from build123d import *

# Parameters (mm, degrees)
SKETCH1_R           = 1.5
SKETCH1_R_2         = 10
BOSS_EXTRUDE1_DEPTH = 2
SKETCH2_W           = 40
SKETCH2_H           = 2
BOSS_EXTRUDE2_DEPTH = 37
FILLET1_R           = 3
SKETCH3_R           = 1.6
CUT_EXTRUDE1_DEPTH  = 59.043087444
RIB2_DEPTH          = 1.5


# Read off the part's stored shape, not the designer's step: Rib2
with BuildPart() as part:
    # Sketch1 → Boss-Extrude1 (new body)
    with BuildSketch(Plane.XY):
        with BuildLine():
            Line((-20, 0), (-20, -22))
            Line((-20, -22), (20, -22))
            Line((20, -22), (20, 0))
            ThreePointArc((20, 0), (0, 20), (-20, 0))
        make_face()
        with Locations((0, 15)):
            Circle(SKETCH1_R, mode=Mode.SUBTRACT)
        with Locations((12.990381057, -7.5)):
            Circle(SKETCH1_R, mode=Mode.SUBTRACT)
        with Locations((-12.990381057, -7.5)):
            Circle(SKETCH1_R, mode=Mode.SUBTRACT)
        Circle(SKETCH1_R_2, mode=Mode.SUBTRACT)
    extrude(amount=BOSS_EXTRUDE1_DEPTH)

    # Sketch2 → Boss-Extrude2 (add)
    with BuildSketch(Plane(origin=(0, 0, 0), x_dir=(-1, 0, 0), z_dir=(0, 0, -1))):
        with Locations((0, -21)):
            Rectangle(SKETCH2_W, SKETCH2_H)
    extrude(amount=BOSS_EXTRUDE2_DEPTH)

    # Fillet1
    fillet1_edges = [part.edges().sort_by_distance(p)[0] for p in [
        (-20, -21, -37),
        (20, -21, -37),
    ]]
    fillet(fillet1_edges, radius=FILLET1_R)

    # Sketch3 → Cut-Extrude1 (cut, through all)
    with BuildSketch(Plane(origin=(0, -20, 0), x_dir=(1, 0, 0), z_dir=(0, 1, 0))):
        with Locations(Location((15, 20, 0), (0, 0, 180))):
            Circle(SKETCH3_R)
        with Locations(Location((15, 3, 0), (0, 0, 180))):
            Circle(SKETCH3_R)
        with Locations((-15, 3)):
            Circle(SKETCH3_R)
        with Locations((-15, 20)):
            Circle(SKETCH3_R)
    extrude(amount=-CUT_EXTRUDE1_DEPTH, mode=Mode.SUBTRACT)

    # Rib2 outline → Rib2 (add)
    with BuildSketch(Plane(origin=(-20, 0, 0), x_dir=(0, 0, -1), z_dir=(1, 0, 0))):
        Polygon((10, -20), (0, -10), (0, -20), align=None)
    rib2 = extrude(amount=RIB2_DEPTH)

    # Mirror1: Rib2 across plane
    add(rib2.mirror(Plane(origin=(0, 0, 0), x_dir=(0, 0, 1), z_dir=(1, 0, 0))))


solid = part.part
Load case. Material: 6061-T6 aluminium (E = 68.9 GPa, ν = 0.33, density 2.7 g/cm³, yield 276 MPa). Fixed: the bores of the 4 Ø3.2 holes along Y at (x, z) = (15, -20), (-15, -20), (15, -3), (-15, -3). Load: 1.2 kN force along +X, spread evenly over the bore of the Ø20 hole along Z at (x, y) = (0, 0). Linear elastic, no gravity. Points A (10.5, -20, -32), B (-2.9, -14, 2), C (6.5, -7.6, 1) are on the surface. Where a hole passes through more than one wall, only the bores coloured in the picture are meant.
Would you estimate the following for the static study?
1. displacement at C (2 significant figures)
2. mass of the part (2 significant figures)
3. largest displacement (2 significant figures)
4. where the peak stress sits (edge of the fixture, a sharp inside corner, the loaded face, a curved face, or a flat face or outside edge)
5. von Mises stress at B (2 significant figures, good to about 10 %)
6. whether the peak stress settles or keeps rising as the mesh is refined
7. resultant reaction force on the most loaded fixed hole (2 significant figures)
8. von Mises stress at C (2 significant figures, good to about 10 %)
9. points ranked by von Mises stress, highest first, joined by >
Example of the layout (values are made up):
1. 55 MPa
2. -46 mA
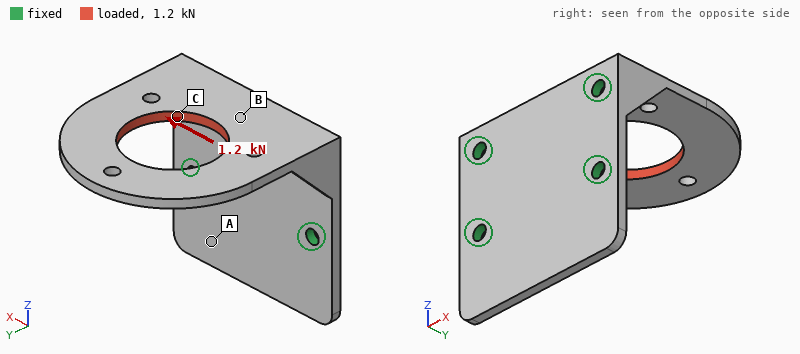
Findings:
1. 0.037 mm
2. 15 g
3. 0.12 mm
4. edge of the fixture
5. 37 MPa
6. keeps rising
7. 990 N
8. 110 MPa
9. C > B > A
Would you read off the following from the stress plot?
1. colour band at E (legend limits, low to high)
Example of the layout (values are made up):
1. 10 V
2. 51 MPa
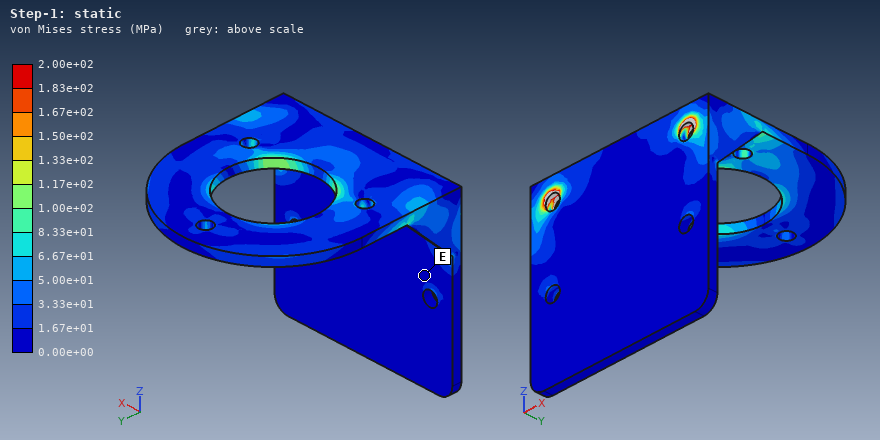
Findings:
1. 0.00e+00 to 1.67e+01 MPa
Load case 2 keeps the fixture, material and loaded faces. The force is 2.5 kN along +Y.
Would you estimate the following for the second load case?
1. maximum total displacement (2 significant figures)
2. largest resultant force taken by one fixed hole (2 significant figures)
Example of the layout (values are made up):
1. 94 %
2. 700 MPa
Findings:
1. 0.27 mm
2. 1.3 kN
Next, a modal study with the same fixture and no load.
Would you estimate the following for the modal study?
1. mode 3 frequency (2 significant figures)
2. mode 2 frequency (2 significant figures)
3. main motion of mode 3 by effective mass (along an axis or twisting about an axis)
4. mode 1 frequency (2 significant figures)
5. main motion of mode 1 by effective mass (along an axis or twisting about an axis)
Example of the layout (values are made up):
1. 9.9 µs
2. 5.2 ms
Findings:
1. 5100 Hz
2. 3500 Hz
3. along Y
4. 1300 Hz
5. along Z
